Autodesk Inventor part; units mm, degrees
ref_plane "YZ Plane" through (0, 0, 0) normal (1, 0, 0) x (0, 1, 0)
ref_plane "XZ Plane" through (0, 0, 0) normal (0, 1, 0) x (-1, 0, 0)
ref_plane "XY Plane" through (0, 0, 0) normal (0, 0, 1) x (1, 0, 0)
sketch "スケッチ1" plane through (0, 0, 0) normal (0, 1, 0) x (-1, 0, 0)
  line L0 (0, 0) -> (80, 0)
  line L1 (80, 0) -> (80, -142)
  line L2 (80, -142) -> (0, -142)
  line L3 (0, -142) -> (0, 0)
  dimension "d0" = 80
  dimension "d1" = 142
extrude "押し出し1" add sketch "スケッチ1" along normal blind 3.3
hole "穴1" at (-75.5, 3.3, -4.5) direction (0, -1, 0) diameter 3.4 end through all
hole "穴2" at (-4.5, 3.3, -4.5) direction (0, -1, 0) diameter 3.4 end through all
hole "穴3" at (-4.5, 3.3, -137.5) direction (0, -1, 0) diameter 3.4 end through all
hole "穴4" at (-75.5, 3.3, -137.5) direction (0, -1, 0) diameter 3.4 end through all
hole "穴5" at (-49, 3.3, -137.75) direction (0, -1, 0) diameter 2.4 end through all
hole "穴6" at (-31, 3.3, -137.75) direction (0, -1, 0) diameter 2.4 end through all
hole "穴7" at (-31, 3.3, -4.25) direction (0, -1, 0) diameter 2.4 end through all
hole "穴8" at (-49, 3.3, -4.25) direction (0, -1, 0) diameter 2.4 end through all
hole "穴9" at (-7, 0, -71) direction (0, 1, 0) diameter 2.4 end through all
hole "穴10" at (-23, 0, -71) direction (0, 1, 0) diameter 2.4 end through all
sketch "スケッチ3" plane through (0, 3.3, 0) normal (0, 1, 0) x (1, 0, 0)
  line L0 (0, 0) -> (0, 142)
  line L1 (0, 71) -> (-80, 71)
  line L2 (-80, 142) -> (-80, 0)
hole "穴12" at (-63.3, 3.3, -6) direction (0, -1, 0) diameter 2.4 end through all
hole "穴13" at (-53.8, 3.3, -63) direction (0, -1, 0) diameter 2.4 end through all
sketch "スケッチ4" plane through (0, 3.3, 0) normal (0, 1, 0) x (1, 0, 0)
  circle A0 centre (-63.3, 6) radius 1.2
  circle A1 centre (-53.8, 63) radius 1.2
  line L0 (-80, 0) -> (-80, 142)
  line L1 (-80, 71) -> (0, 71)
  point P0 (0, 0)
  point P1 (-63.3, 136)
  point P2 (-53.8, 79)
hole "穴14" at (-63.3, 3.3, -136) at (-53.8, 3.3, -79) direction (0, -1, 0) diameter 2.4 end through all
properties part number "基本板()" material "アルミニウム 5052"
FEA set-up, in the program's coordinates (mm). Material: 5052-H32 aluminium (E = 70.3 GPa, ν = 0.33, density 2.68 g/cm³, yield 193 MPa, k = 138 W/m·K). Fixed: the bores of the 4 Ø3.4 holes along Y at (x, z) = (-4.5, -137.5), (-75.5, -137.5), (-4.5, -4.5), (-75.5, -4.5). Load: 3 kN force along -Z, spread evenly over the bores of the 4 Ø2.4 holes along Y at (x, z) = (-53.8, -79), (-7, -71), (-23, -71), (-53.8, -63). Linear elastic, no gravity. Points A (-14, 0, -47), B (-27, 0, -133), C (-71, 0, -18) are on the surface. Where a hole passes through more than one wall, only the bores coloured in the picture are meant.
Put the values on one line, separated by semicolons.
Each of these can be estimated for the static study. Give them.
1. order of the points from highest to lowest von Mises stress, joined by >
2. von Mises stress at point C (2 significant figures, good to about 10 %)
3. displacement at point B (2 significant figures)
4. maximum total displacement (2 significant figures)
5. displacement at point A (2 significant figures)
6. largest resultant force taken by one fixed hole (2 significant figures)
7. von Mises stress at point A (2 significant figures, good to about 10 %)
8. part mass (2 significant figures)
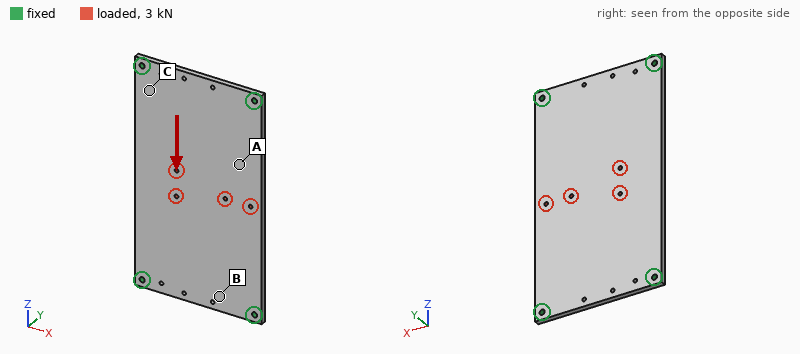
C > A > B; 12 MPa; 6.4 µm; 11 µm; 7.8 µm; 810 N; 7.0 MPa; 100 g
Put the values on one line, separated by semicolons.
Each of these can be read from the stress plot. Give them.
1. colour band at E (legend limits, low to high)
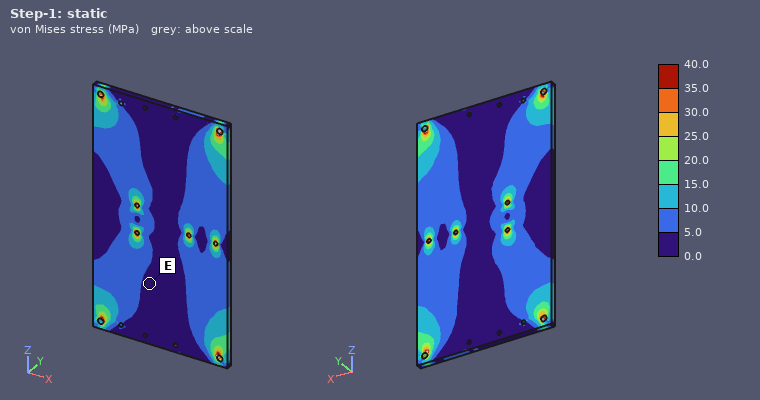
0.0 to 5.0 MPa
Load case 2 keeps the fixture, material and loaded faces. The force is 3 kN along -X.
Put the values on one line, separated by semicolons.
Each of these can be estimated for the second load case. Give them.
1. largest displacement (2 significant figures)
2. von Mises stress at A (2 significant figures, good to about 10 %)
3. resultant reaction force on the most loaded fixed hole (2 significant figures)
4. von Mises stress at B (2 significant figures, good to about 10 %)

25 µm; 9.5 MPa; 1.0 kN; 8.2 MPa
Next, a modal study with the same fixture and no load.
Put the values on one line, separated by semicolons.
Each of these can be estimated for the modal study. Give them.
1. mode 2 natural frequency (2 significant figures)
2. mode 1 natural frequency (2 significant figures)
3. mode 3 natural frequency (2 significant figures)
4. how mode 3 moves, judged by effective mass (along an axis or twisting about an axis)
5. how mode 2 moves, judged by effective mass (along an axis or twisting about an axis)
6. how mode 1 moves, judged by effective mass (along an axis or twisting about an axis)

1400 Hz; 790 Hz; 2200 Hz; twisting about X; twisting about Z; along Y
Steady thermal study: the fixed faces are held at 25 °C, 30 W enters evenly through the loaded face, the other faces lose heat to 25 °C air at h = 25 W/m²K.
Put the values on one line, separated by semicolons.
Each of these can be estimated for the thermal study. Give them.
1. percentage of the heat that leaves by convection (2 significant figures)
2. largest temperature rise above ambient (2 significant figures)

31 %; 33 K
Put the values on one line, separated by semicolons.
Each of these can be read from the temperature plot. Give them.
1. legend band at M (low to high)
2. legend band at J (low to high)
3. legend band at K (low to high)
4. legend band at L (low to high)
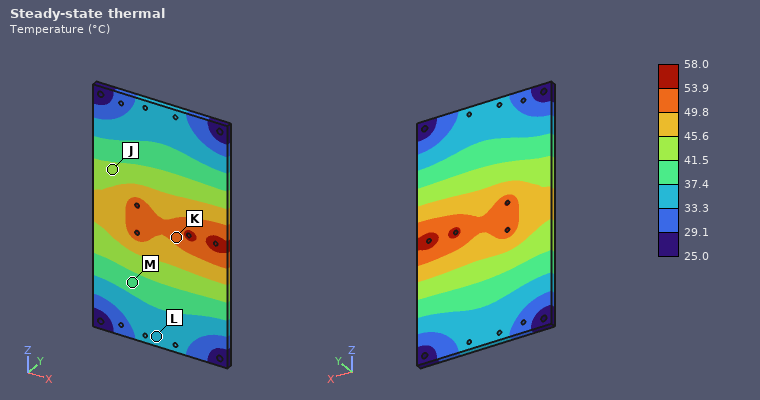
37.4 to 41.5 °C; 41.5 to 45.6 °C; 49.8 to 53.9 °C; 33.3 to 37.4 °C
